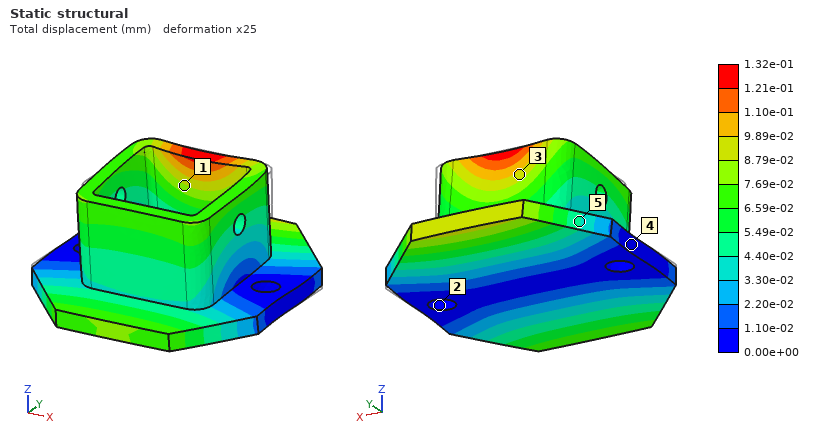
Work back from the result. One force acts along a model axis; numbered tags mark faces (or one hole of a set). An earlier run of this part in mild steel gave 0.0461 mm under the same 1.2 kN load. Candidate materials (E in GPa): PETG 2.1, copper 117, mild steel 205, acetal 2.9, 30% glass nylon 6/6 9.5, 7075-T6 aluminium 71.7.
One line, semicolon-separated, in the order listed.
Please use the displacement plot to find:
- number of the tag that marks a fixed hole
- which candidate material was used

2; 7075-T6 aluminium
